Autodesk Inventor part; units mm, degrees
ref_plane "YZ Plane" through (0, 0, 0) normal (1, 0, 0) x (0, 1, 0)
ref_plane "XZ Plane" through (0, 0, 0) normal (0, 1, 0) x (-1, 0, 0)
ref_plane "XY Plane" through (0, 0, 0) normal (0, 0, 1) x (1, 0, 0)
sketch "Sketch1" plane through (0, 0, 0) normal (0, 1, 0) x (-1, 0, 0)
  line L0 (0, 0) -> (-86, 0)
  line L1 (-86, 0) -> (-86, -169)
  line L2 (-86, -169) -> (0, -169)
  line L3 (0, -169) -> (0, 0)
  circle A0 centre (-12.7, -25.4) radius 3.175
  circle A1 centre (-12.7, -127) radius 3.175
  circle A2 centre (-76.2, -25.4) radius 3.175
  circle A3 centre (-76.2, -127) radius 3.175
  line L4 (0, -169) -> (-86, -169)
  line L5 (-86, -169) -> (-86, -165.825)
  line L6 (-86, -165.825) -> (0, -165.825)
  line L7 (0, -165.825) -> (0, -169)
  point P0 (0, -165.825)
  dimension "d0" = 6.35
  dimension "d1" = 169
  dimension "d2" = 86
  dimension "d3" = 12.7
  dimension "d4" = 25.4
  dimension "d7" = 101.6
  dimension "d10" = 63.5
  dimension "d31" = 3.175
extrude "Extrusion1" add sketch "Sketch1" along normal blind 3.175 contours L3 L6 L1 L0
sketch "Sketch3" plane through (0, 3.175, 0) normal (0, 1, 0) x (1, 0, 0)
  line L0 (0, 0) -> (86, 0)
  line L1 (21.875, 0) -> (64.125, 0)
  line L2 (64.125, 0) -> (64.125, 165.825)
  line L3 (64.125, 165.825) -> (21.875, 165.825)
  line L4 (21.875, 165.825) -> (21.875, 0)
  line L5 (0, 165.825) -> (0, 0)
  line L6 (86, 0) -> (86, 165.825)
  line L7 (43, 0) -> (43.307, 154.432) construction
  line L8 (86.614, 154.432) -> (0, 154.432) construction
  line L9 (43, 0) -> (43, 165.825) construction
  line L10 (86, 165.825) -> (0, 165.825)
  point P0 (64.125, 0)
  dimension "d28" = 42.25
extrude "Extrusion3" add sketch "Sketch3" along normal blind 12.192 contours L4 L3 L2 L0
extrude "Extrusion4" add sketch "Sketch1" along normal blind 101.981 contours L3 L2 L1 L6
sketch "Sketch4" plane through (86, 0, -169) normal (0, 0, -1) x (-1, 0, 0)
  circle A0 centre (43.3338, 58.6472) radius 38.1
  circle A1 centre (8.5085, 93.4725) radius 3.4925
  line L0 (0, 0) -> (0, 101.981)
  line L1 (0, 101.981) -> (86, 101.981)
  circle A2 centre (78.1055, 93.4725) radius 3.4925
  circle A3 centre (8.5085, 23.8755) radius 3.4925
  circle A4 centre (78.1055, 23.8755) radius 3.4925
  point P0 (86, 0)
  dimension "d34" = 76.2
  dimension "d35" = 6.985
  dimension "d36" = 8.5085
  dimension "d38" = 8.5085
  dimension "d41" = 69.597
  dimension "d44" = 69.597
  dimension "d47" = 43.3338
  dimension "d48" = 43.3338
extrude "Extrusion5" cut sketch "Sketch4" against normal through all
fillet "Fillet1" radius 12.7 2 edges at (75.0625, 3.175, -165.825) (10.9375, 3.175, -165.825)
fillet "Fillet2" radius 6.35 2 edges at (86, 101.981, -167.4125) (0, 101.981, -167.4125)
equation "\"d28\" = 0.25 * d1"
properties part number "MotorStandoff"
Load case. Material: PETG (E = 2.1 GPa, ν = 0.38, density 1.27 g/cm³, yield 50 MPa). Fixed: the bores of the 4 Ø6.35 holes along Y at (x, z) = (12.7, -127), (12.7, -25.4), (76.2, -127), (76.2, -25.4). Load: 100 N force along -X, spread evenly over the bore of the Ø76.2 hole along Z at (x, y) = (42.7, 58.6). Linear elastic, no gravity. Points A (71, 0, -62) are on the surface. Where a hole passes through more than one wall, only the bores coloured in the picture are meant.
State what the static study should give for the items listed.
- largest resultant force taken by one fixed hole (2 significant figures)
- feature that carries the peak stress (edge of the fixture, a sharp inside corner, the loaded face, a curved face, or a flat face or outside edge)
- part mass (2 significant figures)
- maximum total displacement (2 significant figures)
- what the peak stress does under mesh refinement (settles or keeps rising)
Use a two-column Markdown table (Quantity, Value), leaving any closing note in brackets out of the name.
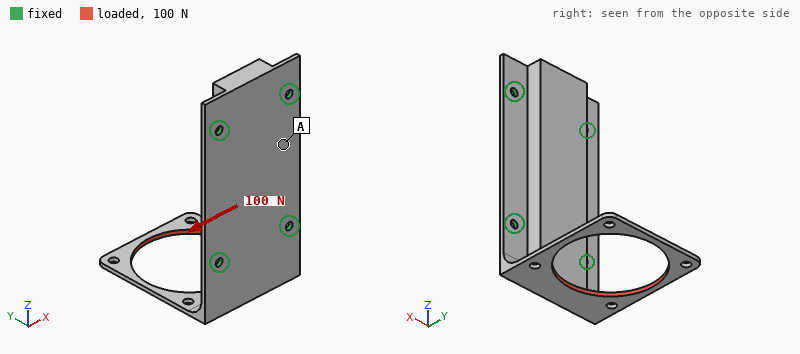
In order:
| Quantity | Value |
|---|---|
| largest resultant force taken by one fixed hole | 120 N |
| feature that carries the peak stress | edge of the fixture |
| part mass | 180 g |
| maximum total displacement | 2.5 mm |
| what the peak stress does under mesh refinement | keeps rising |
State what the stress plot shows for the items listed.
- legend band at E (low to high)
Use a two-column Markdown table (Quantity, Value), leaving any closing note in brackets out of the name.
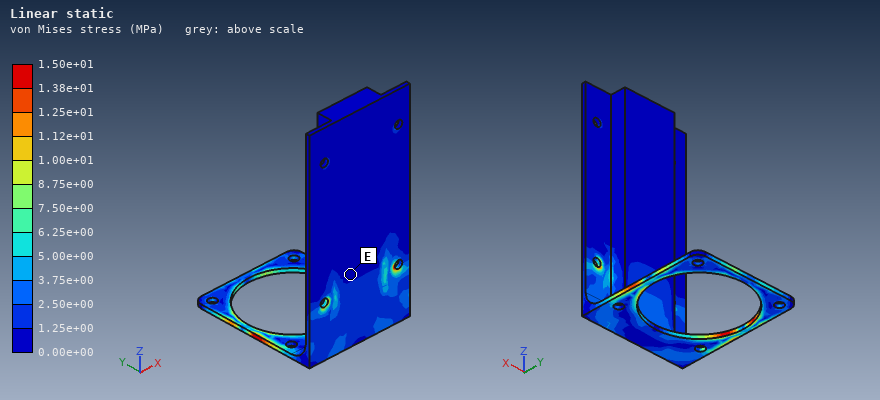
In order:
| Quantity | Value |
|---|---|
| legend band at E | 0.00e+00 to 1.25e+00 MPa |
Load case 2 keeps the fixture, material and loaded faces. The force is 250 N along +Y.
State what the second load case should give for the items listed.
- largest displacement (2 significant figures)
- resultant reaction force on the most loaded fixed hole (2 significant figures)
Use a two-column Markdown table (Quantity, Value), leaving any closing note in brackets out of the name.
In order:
| Quantity | Value |
|---|---|
| largest displacement | 2.5 mm |
| resultant reaction force on the most loaded fixed hole | 300 N |
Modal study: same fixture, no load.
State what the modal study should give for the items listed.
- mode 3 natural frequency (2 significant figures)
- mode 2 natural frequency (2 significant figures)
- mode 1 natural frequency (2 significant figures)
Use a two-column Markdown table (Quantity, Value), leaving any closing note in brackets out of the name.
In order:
| Quantity | Value |
|---|---|
| mode 3 natural frequency | 320 Hz |
| mode 2 natural frequency | 140 Hz |
| mode 1 natural frequency | 60 Hz |
